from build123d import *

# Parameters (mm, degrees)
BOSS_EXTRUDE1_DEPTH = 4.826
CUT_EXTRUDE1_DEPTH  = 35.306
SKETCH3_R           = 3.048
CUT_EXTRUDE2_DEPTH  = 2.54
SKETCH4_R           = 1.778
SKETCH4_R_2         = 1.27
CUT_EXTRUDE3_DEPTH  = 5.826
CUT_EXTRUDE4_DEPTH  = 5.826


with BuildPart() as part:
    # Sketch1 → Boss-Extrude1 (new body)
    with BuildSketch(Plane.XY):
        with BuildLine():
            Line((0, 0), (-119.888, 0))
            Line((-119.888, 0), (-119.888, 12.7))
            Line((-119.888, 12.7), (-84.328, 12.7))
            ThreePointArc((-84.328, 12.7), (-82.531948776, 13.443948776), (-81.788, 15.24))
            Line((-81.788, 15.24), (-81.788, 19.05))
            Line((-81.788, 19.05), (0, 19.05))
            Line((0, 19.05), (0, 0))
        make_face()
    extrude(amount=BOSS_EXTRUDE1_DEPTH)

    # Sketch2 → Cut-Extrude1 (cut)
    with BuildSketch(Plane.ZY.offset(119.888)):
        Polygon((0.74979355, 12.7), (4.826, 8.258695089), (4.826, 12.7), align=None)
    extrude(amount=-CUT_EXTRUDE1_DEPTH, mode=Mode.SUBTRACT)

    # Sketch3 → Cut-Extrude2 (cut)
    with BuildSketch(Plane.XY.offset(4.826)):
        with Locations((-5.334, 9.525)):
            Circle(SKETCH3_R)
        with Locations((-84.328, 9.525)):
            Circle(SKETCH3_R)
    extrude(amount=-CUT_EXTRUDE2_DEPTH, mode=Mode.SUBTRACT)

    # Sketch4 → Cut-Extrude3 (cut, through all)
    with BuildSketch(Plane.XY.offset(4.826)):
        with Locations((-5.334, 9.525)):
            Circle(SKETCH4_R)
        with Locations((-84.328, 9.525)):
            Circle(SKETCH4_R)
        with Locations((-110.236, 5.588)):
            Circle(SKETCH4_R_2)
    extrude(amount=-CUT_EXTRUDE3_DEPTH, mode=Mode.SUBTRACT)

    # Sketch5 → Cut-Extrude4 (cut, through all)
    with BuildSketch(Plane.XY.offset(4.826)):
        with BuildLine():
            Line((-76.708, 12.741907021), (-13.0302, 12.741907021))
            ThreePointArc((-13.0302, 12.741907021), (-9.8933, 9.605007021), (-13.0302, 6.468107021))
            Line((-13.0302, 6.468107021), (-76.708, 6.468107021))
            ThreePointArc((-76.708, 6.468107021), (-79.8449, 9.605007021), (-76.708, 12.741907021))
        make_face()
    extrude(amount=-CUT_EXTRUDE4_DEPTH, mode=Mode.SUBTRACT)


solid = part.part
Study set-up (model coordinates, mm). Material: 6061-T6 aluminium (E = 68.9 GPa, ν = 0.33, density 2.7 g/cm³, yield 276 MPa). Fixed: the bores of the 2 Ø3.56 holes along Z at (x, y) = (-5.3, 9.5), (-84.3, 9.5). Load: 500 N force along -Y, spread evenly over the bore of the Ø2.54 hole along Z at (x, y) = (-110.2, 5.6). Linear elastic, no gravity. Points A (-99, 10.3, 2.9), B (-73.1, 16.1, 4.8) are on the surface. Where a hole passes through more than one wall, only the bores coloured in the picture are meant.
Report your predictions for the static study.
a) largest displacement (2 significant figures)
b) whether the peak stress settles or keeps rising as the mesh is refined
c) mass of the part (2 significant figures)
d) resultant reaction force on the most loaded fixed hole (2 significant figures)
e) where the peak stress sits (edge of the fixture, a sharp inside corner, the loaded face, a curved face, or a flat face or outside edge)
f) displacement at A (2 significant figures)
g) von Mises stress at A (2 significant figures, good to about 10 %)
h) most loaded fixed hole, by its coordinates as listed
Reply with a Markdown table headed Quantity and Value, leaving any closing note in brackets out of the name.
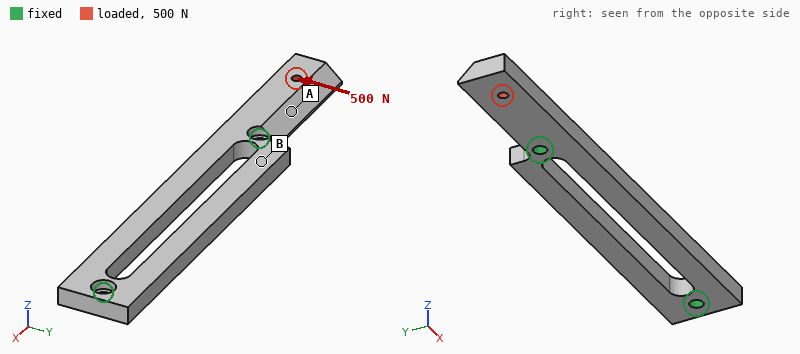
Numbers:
| Quantity | Value |
|---|---|
| largest displacement | 0.31 mm |
| whether the peak stress settles or keeps rising as the mesh is refined | keeps rising |
| mass of the part | 20 g |
| resultant reaction force on the most loaded fixed hole | 670 N |
| where the peak stress sits | edge of the fixture |
| displacement at A | 0.10 mm |
| von Mises stress at A | 54 MPa |
| most loaded fixed hole, by its coordinates as listed | (-84.3, 9.5) |
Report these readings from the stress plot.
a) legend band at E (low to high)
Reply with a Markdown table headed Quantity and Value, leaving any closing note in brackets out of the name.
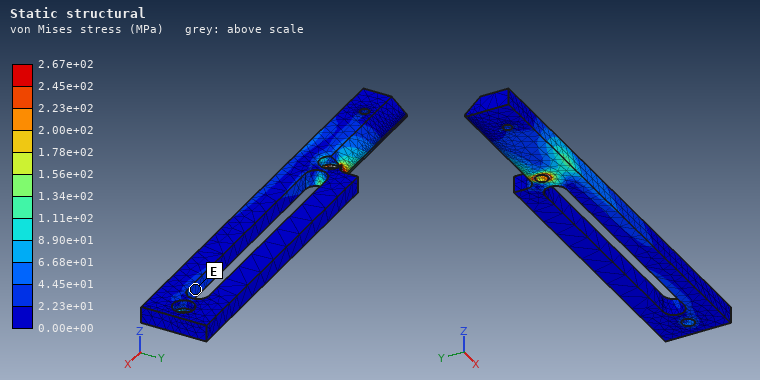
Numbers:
| Quantity | Value |
|---|---|
| legend band at E | 2.23e+01 to 4.45e+01 MPa |
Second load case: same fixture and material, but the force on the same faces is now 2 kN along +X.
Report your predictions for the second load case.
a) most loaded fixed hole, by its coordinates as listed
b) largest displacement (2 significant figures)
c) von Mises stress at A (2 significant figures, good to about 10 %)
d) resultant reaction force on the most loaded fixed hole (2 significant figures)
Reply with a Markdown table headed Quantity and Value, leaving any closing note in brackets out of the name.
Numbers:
| Quantity | Value |
|---|---|
| most loaded fixed hole, by its coordinates as listed | (-84.3, 9.5) |
| largest displacement | 0.14 mm |
| von Mises stress at A | 44 MPa |
| resultant reaction force on the most loaded fixed hole | 1.7 kN |
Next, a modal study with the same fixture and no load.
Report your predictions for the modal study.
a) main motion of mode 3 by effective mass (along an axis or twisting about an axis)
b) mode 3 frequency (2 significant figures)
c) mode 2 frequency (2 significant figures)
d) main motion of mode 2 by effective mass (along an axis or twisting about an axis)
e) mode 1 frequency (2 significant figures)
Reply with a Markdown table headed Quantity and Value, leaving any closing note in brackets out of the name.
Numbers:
| Quantity | Value |
|---|---|
| main motion of mode 3 by effective mass | along Z |
| mode 3 frequency | 3500 Hz |
| mode 2 frequency | 3100 Hz |
| main motion of mode 2 by effective mass | along Z |
| mode 1 frequency | 2200 Hz |
